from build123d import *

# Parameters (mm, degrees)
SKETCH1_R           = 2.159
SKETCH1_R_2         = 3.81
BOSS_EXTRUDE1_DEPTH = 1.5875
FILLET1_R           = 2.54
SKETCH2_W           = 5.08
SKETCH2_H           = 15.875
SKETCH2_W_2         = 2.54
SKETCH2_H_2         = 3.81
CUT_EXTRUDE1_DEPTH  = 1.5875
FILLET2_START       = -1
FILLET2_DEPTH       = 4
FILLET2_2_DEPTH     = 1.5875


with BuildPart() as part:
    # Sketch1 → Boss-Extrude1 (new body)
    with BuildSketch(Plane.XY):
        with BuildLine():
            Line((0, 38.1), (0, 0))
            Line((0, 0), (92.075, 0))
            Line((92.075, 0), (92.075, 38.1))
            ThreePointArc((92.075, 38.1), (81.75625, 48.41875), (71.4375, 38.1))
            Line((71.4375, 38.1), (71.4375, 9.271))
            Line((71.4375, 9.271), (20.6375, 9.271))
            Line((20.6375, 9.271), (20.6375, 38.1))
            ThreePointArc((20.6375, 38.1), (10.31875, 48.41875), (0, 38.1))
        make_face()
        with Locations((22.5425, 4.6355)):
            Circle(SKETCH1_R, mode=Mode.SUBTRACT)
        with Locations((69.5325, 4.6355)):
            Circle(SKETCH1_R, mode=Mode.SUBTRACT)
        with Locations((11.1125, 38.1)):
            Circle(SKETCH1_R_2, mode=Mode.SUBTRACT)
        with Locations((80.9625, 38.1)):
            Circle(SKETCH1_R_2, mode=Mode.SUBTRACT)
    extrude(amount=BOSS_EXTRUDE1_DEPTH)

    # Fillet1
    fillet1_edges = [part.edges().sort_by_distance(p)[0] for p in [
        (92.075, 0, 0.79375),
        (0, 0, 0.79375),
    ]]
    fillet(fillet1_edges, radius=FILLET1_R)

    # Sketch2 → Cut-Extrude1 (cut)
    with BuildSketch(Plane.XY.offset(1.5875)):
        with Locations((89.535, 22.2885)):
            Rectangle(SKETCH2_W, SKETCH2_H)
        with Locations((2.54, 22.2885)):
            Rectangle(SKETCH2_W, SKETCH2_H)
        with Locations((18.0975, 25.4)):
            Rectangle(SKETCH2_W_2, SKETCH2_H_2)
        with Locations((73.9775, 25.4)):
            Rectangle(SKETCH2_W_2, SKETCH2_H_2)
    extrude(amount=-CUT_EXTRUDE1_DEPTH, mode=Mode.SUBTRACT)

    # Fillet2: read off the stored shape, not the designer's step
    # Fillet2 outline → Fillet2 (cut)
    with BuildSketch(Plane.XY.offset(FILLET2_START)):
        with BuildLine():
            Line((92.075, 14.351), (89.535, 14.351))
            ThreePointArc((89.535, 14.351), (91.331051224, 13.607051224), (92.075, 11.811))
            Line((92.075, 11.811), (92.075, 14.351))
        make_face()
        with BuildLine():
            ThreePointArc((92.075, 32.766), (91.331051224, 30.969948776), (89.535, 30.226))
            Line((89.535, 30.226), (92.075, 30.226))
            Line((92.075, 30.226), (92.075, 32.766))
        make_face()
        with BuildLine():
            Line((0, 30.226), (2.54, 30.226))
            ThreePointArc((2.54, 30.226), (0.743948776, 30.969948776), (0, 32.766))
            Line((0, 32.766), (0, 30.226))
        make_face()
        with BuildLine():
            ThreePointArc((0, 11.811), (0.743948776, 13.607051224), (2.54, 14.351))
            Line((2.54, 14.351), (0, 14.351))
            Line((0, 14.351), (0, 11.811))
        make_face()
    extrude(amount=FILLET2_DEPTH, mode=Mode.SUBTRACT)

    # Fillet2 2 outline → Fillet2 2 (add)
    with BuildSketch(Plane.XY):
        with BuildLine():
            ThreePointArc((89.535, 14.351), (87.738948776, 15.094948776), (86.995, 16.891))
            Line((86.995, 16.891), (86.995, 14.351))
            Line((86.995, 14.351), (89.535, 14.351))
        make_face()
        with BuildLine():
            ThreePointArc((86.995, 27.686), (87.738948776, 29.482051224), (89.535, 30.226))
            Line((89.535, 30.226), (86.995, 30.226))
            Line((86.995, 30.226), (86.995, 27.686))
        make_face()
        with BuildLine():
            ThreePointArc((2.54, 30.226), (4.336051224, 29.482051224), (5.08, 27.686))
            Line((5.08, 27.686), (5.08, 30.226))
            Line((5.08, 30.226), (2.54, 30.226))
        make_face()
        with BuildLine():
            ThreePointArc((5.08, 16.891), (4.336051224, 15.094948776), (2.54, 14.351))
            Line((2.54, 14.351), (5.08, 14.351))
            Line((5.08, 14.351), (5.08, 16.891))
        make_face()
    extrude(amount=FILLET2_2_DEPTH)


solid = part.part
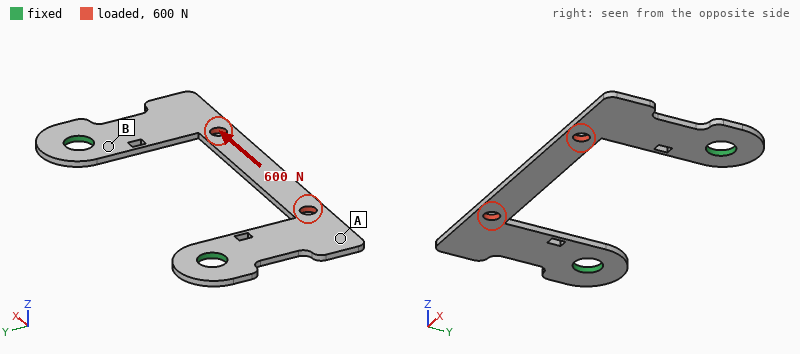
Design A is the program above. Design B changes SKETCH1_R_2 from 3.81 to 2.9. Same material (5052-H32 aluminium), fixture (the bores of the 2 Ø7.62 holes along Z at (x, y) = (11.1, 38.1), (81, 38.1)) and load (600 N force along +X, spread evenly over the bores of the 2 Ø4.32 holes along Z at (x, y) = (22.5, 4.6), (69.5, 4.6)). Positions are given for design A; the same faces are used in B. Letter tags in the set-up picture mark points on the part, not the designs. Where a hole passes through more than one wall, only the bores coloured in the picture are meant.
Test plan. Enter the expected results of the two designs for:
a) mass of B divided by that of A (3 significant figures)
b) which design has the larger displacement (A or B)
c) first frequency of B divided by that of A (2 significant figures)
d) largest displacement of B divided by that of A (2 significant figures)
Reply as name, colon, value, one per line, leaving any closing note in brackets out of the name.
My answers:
mass of B divided by that of A: 1.02
which design has the larger displacement: B
first frequency of B divided by that of A: 0.96
largest displacement of B divided by that of A: 1.2
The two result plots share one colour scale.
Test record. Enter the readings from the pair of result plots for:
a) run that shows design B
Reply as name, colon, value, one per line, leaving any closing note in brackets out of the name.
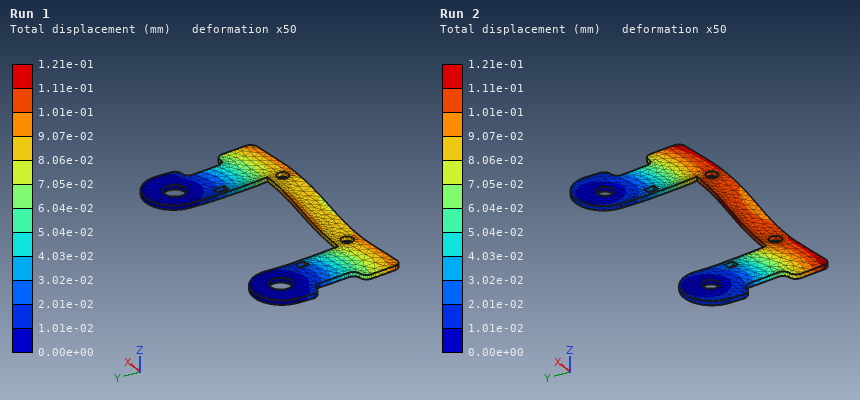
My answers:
run that shows design B: Run 2
